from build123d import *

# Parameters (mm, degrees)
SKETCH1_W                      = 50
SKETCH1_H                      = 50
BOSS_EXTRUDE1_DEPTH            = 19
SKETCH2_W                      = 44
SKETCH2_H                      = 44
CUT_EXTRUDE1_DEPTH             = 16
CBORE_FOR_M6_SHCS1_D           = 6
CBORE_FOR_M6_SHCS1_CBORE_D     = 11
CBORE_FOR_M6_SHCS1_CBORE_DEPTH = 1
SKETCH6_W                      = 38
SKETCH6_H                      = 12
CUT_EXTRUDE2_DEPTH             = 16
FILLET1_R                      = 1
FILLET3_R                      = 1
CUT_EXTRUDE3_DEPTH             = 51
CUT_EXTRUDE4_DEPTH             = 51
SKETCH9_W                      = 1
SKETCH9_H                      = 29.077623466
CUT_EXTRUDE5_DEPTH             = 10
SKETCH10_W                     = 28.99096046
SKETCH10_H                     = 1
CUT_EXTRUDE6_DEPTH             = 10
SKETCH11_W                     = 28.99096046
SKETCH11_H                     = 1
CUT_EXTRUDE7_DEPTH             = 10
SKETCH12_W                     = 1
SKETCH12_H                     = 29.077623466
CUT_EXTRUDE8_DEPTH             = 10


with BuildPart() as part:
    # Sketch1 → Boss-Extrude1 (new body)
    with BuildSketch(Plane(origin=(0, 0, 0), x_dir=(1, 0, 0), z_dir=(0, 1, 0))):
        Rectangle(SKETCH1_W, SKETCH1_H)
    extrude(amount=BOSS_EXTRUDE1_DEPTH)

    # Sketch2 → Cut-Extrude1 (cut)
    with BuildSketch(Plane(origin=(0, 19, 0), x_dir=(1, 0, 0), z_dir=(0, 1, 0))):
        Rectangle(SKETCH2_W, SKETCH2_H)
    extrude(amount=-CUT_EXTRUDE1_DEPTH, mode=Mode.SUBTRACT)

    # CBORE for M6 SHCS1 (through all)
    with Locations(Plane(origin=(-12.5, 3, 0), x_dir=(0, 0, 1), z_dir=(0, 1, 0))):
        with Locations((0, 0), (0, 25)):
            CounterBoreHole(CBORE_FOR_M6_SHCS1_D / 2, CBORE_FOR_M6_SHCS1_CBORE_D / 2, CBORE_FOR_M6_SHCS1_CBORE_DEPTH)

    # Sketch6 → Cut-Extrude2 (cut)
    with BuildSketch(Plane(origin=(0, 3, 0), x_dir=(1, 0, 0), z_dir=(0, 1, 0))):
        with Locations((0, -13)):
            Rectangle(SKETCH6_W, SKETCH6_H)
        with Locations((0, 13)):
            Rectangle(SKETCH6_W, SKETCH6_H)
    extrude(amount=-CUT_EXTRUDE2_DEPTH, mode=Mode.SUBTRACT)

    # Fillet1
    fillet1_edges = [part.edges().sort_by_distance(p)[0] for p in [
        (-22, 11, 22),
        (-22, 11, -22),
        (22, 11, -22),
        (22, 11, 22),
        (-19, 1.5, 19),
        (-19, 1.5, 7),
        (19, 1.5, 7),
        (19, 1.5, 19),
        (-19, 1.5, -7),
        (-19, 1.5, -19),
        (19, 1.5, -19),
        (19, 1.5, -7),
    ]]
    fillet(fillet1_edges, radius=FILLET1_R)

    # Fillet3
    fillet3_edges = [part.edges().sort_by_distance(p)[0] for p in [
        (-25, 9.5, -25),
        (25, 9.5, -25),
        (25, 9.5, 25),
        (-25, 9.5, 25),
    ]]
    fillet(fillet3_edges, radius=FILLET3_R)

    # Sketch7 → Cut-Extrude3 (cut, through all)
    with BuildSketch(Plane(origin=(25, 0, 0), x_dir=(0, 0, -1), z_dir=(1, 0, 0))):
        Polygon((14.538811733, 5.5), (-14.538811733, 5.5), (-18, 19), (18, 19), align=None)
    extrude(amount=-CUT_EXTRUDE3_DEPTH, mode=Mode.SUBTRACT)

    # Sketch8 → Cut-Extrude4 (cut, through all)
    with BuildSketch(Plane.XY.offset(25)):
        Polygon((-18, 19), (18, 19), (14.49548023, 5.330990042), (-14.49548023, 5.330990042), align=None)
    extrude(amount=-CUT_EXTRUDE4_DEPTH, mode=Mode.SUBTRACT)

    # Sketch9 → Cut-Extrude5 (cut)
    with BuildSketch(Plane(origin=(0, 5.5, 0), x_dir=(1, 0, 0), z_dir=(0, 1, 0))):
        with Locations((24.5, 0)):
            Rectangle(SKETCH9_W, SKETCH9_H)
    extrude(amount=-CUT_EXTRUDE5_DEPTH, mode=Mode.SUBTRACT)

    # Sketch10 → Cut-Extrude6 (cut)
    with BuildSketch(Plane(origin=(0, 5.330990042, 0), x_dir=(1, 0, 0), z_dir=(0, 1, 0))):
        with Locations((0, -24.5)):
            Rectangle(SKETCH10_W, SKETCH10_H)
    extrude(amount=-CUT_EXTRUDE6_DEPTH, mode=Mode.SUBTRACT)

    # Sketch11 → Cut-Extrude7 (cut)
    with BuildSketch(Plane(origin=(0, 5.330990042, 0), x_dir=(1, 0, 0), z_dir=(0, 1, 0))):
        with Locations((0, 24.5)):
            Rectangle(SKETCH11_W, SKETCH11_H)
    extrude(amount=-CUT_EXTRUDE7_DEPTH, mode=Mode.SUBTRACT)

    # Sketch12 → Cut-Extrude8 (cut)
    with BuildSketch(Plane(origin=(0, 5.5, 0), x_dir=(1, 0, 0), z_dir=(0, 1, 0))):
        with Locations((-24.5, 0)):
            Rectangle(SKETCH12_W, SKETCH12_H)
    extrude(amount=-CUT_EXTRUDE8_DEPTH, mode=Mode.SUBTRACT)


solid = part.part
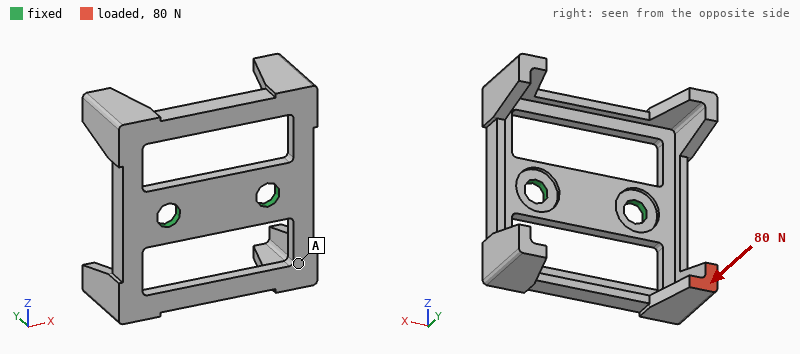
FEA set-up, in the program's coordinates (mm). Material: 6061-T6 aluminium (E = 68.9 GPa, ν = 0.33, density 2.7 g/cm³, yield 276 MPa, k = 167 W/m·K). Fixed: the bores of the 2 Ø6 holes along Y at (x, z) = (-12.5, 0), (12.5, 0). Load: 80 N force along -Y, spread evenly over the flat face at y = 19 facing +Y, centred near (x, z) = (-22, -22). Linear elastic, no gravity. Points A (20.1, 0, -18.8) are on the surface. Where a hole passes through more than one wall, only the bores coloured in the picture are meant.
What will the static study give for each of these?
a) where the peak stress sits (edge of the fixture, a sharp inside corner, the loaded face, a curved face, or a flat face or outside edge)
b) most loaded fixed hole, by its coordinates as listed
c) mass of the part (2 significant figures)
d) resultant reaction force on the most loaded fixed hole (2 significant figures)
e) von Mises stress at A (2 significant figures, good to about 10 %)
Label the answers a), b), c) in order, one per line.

a) a flat face or outside edge
b) (-12.5, 0)
c) 20 g
d) 89 N
e) 8.5 MPa
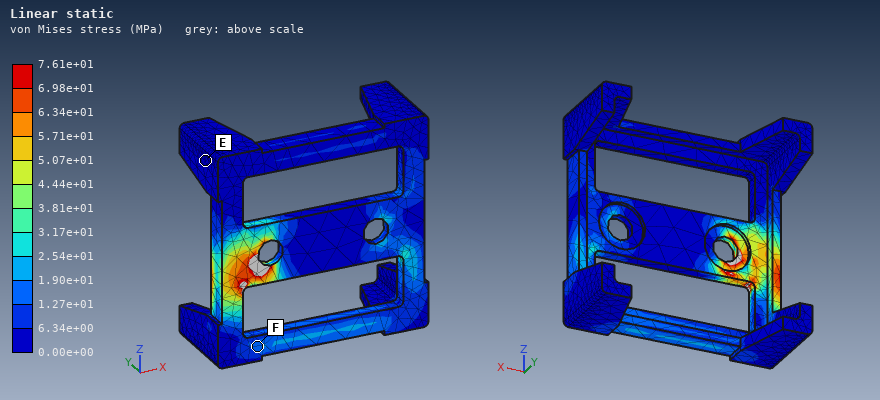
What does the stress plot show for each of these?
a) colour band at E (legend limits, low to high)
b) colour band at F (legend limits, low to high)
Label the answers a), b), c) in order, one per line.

a) 0.00e+00 to 6.34e+00 MPa
b) 1.27e+01 to 1.90e+01 MPa
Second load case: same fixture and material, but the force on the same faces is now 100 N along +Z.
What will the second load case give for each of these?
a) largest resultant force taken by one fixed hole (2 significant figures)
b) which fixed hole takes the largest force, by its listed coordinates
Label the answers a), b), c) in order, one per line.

a) 110 N
b) (-12.5, 0)
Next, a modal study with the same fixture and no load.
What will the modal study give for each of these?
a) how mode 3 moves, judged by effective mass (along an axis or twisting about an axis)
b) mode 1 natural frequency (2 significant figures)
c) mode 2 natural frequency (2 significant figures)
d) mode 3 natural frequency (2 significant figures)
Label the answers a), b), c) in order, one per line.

a) along Y
b) 1400 Hz
c) 1900 Hz
d) 2300 Hz
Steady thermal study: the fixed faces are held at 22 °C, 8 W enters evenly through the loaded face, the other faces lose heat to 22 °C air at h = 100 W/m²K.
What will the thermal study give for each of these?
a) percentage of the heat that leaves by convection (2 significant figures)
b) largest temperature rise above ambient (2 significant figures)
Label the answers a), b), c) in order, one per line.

a) 47 %
b) 37 K
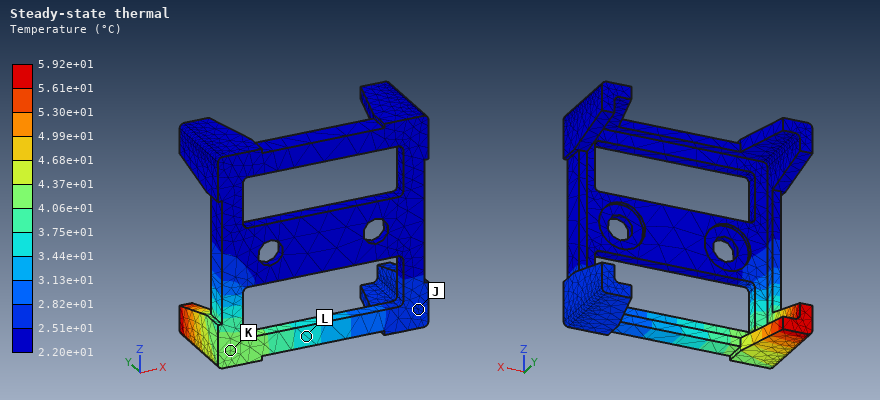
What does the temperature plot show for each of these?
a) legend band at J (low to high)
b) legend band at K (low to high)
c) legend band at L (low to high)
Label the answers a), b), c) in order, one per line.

a) 2.51e+01 to 2.82e+01 °C
b) 4.06e+01 to 4.37e+01 °C
c) 3.44e+01 to 3.75e+01 °C
